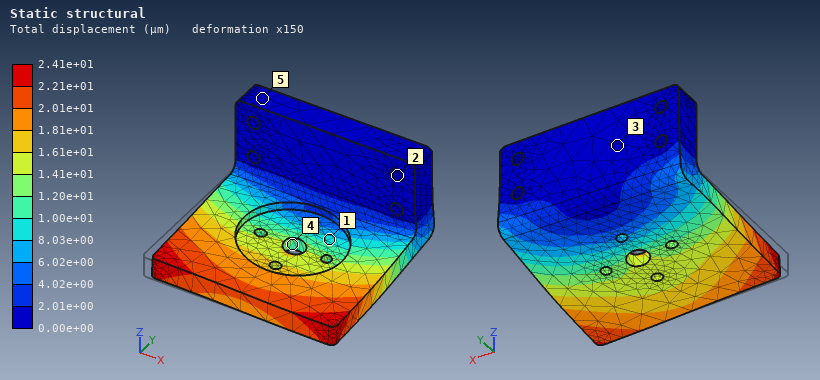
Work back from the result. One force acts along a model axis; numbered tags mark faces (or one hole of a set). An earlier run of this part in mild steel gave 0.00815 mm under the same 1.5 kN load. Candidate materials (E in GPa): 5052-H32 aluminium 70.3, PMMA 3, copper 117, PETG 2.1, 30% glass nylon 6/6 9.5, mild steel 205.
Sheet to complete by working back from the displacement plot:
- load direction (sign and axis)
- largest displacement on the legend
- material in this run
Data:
+X
2.41e+01 µm
5052-H32 aluminium
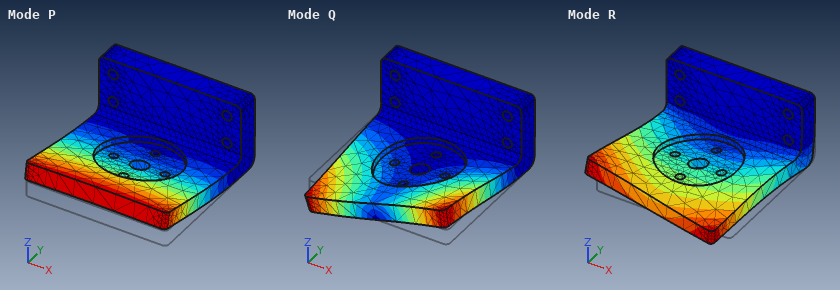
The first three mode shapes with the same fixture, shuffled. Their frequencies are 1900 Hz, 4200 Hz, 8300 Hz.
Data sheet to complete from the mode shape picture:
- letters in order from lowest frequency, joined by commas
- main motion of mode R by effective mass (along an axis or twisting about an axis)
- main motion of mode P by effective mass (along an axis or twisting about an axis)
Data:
P, Q, R
along X
along Z
